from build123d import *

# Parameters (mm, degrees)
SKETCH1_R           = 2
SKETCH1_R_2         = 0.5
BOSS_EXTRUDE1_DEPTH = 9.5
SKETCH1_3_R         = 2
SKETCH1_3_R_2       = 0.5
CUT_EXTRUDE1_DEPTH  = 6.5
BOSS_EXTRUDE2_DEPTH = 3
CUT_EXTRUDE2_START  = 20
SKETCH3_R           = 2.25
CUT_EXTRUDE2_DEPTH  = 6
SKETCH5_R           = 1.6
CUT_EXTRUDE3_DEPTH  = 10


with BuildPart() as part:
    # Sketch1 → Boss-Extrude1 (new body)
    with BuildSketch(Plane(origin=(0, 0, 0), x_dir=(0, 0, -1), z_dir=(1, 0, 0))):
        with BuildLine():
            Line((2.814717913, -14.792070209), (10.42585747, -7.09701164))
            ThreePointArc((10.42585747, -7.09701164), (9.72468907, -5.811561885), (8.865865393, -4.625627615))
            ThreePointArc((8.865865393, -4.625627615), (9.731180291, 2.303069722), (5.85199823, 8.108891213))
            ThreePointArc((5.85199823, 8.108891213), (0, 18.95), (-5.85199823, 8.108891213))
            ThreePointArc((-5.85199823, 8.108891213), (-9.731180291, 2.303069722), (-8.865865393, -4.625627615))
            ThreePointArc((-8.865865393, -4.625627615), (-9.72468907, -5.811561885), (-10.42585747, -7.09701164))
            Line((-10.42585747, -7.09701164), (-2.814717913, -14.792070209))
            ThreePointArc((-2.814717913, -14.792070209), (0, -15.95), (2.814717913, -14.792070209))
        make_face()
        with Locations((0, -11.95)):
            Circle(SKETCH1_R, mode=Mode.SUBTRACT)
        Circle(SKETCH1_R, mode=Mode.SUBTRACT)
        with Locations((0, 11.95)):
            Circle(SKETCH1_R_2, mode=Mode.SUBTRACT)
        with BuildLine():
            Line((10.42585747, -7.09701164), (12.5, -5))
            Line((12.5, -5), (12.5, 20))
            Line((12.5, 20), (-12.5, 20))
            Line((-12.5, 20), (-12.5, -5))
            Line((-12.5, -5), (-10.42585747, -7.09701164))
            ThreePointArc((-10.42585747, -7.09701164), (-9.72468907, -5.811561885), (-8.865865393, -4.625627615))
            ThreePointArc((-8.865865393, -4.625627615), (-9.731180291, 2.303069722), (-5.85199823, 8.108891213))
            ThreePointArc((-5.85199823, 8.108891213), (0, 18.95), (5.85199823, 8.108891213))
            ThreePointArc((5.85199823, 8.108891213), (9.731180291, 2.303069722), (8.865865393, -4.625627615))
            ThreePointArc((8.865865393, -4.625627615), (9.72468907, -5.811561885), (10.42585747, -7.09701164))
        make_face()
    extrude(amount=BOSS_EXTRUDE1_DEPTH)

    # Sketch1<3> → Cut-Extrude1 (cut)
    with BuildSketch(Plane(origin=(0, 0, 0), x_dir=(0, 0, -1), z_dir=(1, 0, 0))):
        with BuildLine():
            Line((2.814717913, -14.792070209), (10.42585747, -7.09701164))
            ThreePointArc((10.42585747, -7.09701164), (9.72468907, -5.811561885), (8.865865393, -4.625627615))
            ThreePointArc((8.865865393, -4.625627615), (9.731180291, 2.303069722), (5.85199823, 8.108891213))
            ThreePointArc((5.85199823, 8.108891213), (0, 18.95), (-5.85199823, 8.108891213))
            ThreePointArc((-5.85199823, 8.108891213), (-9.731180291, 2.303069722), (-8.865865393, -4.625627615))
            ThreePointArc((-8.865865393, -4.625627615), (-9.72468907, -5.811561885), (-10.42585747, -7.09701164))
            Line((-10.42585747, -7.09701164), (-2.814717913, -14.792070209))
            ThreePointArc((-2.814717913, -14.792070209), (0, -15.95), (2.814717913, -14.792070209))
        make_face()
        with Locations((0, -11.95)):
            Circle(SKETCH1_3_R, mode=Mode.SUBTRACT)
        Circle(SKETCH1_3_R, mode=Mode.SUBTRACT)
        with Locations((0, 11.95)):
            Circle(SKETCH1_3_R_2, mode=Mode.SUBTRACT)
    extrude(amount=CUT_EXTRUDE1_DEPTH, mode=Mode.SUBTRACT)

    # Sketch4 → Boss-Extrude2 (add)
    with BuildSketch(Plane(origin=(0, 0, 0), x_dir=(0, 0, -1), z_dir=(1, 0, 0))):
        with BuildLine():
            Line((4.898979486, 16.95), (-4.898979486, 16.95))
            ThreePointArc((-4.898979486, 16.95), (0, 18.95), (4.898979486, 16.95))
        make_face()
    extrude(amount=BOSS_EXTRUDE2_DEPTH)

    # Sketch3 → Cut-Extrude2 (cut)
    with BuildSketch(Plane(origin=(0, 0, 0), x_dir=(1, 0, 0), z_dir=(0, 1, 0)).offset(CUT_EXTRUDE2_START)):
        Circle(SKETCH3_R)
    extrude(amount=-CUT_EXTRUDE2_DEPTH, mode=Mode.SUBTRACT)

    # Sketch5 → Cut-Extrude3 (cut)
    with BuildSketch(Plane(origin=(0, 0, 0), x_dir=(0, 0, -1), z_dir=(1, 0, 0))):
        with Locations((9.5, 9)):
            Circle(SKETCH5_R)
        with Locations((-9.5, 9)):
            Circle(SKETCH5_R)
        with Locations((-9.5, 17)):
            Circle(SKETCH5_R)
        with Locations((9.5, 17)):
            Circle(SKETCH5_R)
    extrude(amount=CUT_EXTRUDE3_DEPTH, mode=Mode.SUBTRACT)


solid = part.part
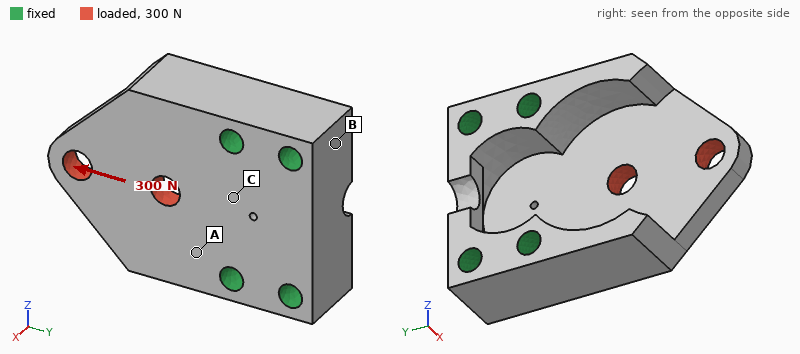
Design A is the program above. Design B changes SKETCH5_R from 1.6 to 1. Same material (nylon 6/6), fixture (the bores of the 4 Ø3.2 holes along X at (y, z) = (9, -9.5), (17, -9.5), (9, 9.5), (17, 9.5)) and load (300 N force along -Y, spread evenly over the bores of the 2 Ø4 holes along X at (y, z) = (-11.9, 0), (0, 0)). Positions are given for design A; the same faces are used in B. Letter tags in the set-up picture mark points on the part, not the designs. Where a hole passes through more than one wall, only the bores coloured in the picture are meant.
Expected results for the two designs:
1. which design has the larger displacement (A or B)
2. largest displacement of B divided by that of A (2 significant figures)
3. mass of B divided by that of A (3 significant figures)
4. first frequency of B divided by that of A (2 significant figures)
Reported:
B
1.1
1.05
0.97
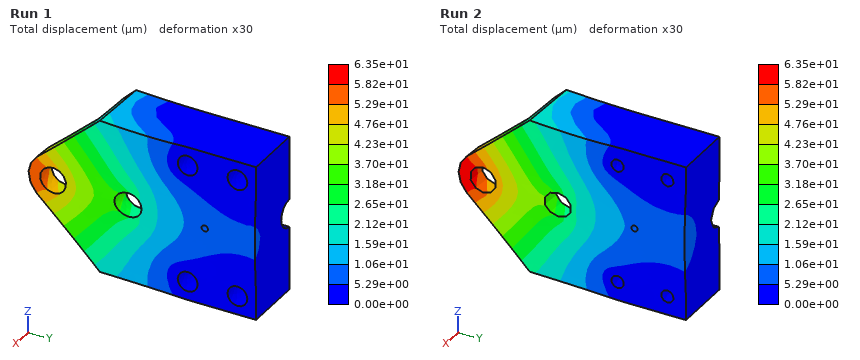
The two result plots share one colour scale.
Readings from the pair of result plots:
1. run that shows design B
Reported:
Run 2
